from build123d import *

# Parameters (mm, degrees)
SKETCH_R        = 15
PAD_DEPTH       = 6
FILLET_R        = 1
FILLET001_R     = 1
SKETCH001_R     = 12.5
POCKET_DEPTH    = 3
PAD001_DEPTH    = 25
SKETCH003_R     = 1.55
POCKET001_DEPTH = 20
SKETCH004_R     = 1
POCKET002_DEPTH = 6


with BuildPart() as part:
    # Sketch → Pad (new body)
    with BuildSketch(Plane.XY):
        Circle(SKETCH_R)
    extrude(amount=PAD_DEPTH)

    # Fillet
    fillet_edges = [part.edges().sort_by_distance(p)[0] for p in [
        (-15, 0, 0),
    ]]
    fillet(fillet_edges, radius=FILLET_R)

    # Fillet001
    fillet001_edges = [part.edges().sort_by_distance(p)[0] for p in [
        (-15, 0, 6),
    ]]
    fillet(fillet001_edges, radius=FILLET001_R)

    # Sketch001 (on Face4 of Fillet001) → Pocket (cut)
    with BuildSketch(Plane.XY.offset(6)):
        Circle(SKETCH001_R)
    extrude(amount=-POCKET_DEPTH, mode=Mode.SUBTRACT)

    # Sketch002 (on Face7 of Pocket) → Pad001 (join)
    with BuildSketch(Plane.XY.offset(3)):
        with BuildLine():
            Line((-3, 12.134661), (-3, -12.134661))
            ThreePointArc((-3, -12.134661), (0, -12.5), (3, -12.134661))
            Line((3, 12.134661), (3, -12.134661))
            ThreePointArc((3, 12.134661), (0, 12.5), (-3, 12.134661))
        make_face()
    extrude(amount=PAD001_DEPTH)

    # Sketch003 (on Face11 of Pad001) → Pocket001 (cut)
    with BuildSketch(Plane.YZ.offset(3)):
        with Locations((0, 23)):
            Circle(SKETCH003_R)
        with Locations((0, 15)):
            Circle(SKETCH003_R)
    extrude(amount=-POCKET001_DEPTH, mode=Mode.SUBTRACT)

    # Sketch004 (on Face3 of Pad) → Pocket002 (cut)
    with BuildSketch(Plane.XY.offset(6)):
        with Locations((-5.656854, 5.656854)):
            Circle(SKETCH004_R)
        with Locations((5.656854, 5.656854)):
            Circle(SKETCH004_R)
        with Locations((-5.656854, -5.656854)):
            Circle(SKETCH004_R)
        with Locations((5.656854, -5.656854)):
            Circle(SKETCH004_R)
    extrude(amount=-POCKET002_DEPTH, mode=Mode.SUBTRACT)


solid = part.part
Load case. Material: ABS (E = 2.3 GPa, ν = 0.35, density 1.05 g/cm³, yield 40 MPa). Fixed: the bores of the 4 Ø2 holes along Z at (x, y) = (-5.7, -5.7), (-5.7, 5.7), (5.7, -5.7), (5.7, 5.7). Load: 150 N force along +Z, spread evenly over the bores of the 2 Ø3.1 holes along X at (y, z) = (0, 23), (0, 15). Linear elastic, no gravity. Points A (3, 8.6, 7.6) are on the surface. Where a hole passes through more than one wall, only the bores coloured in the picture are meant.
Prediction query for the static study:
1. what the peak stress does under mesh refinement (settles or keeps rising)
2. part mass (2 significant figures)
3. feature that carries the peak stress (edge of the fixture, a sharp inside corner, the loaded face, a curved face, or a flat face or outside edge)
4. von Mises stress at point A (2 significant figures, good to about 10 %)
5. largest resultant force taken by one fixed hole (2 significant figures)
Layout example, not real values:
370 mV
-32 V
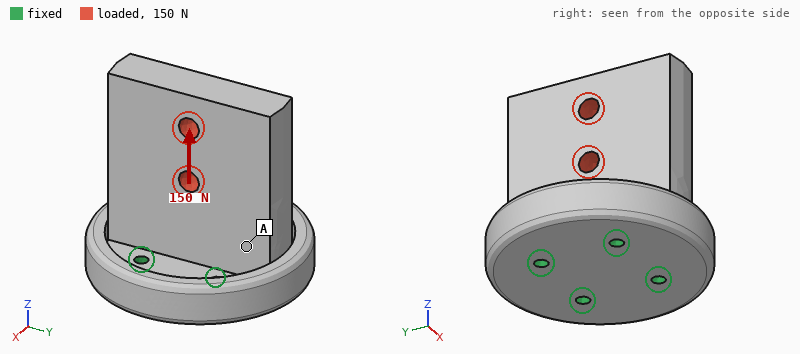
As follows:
keeps rising
6.6 g
edge of the fixture
0.92 MPa
39 N
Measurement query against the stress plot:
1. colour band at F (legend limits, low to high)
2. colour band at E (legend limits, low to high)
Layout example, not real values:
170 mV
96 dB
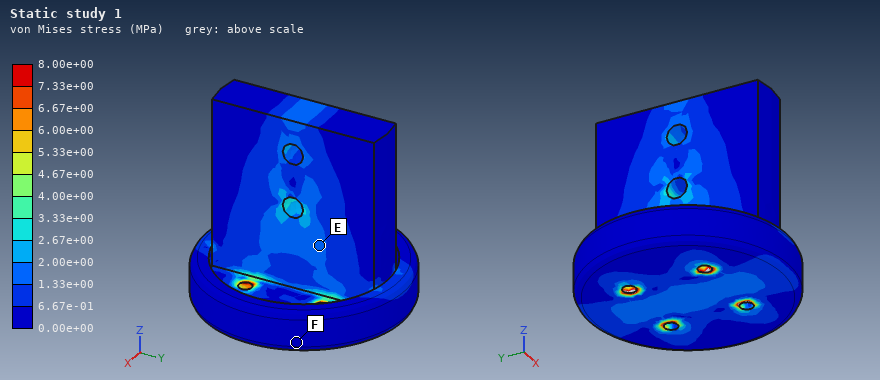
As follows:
0.00e+00 to 6.67e-01 MPa
1.33e+00 to 2.00e+00 MPa
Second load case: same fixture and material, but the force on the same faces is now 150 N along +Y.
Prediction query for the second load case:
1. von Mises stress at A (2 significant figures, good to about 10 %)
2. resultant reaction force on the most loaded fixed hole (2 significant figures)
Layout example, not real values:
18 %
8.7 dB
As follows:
2.1 MPa
100 N
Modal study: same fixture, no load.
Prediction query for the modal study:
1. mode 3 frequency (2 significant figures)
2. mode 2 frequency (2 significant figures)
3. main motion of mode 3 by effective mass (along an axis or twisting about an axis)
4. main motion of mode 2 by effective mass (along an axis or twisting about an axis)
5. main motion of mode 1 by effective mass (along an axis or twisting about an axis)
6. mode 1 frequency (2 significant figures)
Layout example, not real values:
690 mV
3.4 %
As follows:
4300 Hz
3100 Hz
twisting about Z
along Y
along X
1900 Hz
